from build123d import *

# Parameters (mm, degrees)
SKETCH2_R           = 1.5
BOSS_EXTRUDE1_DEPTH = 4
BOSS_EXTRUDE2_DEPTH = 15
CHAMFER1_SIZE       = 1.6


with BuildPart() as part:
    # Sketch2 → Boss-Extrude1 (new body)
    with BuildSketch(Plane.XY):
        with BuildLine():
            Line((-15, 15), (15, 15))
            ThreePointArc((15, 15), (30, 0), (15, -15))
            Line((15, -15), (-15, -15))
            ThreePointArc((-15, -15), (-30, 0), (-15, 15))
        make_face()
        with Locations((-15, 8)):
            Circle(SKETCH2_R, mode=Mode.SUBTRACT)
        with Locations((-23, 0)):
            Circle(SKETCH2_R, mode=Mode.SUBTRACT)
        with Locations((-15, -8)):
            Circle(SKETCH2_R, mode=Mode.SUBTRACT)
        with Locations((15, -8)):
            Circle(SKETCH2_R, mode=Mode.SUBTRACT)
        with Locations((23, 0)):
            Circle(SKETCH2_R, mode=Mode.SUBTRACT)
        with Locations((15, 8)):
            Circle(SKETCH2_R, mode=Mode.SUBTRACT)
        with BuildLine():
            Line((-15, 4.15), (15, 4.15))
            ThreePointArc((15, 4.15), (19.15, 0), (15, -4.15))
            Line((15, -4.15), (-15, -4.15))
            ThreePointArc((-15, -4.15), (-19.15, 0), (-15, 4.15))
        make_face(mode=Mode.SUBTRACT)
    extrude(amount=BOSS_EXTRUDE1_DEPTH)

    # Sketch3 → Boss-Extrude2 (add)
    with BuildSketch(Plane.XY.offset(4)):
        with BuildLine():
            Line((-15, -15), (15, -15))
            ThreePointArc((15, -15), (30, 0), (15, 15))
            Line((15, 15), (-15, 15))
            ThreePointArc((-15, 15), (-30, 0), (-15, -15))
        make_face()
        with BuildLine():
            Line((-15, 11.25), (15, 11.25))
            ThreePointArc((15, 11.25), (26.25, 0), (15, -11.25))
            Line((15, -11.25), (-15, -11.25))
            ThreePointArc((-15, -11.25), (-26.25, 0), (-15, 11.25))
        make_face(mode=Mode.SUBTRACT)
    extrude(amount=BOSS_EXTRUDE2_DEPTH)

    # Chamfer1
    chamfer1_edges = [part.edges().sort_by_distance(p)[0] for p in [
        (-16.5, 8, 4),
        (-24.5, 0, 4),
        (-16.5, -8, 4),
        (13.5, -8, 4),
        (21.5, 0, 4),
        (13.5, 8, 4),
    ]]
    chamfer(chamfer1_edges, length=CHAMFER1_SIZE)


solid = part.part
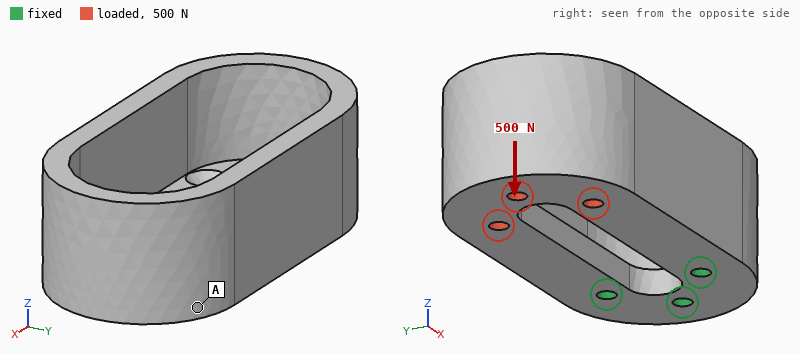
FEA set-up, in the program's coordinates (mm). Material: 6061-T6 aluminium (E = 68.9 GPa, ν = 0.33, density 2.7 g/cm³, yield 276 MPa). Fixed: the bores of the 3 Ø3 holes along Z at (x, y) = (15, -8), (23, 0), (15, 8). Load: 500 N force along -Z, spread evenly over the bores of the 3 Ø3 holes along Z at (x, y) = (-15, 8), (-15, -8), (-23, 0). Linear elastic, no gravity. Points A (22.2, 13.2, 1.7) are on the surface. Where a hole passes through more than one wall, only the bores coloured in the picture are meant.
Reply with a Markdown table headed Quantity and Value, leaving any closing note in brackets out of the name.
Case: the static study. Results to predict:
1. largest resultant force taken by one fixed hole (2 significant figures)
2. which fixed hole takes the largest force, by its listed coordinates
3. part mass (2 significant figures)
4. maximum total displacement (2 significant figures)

| Quantity | Value |
|---|---|
| largest resultant force taken by one fixed hole | 1.2 kN |
| which fixed hole takes the largest force, by its listed coordinates | (23, 0) |
| part mass | 35 g |
| maximum total displacement | 0.15 mm |
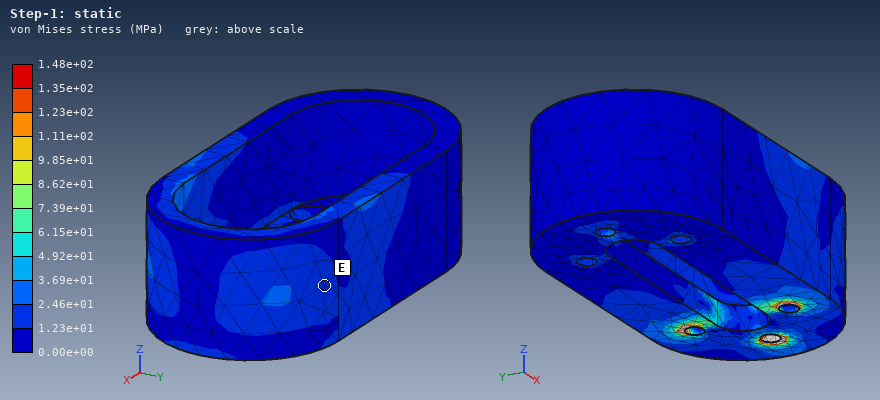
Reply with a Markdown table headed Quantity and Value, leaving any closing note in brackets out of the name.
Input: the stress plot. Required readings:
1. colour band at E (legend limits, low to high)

| Quantity | Value |
|---|---|
| colour band at E | 1.23e+01 to 2.46e+01 MPa |
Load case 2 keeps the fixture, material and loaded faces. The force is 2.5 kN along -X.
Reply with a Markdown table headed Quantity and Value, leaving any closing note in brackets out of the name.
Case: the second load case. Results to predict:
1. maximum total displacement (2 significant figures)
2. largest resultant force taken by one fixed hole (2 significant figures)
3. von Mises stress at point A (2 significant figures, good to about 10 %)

| Quantity | Value |
|---|---|
| maximum total displacement | 40 µm |
| largest resultant force taken by one fixed hole | 1.2 kN |
| von Mises stress at point A | 11 MPa |
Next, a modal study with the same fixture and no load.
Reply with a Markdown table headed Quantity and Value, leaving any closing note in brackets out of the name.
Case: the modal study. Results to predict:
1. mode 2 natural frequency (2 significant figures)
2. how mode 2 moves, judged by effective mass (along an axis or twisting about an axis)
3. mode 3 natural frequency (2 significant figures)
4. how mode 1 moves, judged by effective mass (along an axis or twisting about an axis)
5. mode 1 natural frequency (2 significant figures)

| Quantity | Value |
|---|---|
| mode 2 natural frequency | 3100 Hz |
| how mode 2 moves, judged by effective mass | along Y |
| mode 3 natural frequency | 6000 Hz |
| how mode 1 moves, judged by effective mass | along Z |
| mode 1 natural frequency | 2600 Hz |
